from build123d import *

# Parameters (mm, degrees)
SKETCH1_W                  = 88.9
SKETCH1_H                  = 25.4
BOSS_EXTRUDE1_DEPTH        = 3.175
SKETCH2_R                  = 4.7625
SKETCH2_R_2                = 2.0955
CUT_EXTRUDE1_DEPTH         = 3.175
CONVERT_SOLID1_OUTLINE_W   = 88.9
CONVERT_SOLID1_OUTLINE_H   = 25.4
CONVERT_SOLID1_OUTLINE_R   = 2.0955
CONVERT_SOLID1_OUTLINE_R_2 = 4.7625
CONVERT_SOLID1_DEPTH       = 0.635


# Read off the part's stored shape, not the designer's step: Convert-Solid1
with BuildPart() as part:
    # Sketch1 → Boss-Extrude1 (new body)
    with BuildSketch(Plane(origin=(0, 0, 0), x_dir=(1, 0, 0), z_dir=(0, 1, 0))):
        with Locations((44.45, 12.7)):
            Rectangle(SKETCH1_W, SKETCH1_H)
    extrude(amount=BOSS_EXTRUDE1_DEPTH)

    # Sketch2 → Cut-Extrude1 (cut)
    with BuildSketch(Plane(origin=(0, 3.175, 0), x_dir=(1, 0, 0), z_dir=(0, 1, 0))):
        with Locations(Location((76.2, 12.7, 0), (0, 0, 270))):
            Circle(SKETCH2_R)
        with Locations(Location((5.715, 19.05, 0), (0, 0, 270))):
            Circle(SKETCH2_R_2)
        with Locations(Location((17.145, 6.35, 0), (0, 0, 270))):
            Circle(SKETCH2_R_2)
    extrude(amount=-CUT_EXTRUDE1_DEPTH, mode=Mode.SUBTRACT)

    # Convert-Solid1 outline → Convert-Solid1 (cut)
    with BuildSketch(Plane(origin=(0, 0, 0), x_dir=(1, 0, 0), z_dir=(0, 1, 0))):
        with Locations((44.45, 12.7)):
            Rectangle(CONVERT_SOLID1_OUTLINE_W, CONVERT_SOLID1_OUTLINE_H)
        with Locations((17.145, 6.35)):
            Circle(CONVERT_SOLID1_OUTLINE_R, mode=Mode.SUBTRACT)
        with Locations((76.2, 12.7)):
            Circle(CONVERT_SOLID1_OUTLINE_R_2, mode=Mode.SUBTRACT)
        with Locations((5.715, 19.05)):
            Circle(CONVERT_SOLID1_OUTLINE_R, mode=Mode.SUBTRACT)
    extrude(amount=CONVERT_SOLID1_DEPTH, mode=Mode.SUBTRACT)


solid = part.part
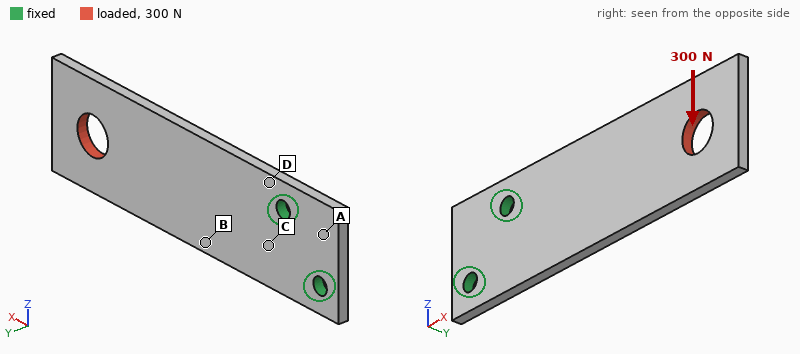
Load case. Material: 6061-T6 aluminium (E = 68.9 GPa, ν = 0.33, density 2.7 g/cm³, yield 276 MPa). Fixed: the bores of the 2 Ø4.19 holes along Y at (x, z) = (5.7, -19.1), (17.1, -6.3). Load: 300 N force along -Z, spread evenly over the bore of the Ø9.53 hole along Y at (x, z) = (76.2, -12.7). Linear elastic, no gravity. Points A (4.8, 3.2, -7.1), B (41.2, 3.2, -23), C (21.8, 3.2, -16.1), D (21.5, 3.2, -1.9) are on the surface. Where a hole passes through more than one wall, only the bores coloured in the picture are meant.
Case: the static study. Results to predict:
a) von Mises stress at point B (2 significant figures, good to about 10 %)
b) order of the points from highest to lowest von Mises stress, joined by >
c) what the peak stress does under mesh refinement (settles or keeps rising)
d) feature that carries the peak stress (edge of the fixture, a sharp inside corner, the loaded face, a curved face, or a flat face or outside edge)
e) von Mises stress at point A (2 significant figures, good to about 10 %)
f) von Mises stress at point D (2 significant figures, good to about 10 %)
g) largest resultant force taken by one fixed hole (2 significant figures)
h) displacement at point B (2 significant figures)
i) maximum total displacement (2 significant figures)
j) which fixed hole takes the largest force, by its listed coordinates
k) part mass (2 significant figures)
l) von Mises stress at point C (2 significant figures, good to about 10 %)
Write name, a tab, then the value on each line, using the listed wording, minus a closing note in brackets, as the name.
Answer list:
von Mises stress at point B	32 MPa
order of the points from highest to lowest von Mises stress, joined by >	D > B > C > A
what the peak stress does under mesh refinement	keeps rising
feature that carries the peak stress	edge of the fixture
von Mises stress at point A	6.3 MPa
von Mises stress at point D	47 MPa
largest resultant force taken by one fixed hole	1.1 kN
displacement at point B	0.042 mm
maximum total displacement	0.17 mm
which fixed hole takes the largest force, by its listed coordinates	(17.1, -6.3)
part mass	15 g
von Mises stress at point C	23 MPa
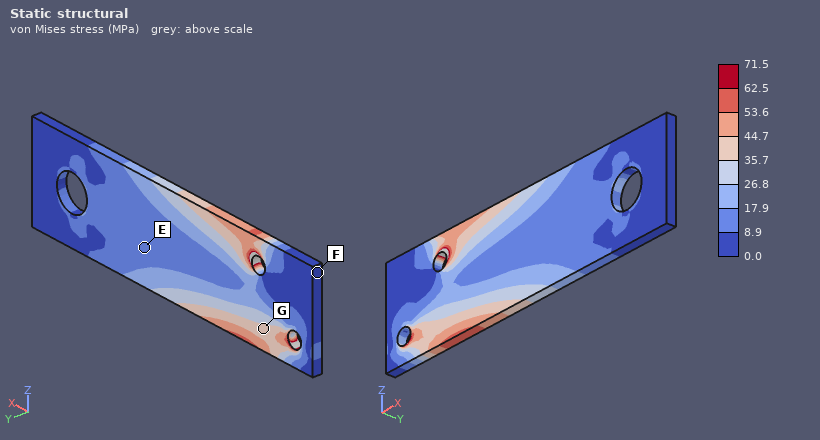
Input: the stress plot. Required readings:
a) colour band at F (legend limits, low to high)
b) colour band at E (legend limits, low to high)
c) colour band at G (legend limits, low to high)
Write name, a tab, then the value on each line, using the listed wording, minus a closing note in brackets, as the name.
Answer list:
colour band at F	0.0 to 8.9 MPa
colour band at E	8.9 to 17.9 MPa
colour band at G	35.7 to 44.7 MPa
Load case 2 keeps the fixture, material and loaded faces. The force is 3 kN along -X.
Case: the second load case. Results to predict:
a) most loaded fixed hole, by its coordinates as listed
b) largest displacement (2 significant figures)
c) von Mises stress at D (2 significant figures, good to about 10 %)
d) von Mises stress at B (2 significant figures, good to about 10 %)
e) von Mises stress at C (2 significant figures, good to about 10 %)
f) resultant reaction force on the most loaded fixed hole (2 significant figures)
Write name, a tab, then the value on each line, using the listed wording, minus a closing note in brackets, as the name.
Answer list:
most loaded fixed hole, by its coordinates as listed	(17.1, -6.3)
largest displacement	63 µm
von Mises stress at D	32 MPa
von Mises stress at B	47 MPa
von Mises stress at C	41 MPa
resultant reaction force on the most loaded fixed hole	1.7 kN
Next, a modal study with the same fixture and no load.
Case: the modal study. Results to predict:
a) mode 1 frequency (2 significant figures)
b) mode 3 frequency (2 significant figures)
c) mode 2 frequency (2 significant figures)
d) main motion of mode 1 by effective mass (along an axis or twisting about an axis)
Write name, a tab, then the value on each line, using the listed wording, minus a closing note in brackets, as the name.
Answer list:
mode 1 frequency	420 Hz
mode 3 frequency	2500 Hz
mode 2 frequency	2100 Hz
main motion of mode 1 by effective mass	along Y
